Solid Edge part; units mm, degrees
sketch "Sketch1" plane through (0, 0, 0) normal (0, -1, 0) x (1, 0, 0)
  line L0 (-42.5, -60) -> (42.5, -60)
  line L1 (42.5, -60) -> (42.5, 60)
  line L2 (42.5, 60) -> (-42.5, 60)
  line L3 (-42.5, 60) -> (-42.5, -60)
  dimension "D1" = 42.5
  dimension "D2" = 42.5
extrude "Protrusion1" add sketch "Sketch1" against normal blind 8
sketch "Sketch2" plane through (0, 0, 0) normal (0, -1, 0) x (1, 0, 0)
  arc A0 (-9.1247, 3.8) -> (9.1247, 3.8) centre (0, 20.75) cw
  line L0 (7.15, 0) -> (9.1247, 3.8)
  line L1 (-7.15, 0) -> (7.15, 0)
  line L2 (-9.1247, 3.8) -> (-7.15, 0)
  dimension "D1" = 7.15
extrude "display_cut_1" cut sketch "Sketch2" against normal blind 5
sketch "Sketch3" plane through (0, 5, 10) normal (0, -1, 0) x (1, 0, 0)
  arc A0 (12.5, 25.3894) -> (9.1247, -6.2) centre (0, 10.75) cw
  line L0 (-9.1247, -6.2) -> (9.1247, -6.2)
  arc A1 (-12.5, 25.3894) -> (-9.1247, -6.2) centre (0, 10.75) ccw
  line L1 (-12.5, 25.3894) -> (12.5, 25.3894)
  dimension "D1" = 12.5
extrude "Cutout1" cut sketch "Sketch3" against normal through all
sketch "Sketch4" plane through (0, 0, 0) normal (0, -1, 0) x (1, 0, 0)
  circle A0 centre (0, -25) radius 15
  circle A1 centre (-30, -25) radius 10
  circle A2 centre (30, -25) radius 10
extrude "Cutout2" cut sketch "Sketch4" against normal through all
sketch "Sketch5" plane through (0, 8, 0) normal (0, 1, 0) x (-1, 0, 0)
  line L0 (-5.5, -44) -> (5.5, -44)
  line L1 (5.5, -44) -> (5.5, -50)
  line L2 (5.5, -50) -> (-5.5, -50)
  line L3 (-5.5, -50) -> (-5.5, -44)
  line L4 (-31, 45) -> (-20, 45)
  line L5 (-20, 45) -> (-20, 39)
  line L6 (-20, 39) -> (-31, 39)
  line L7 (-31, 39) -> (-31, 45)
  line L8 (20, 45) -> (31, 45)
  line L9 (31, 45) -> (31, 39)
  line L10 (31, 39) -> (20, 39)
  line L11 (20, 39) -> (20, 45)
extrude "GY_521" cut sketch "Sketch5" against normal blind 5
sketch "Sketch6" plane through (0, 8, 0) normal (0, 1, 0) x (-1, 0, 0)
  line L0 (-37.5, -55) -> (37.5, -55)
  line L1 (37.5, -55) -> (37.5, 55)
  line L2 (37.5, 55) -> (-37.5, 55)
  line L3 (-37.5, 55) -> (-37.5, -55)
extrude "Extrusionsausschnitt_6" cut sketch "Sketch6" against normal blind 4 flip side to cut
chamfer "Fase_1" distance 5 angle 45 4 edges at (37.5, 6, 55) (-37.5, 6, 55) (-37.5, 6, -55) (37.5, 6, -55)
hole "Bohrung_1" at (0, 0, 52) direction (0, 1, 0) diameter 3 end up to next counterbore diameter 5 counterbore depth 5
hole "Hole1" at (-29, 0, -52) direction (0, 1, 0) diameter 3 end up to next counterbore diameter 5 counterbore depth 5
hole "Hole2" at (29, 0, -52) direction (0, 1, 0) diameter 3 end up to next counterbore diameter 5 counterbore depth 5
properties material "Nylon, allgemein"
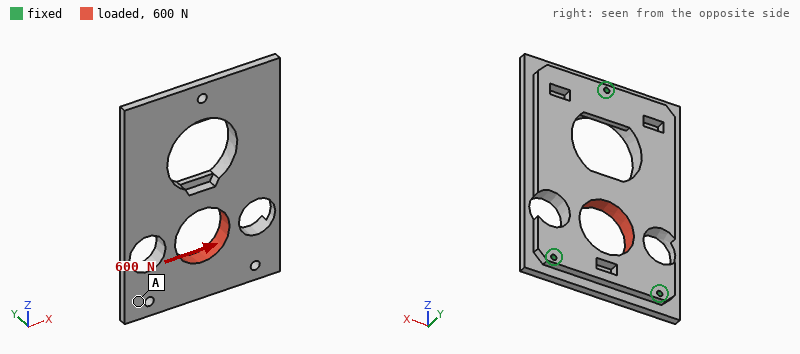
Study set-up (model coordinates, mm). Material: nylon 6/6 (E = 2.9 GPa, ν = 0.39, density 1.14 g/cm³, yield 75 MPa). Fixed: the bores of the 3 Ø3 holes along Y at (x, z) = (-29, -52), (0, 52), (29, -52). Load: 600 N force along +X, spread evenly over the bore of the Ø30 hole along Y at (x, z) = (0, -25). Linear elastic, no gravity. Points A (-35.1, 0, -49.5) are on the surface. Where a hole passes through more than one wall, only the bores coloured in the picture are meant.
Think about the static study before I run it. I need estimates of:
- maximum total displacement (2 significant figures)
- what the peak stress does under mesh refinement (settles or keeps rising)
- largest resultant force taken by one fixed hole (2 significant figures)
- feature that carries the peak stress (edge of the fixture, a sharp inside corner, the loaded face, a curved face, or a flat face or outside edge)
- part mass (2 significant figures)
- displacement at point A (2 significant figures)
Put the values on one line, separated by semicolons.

0.13 mm; keeps rising; 250 N; edge of the fixture; 60 g; 0.029 mm
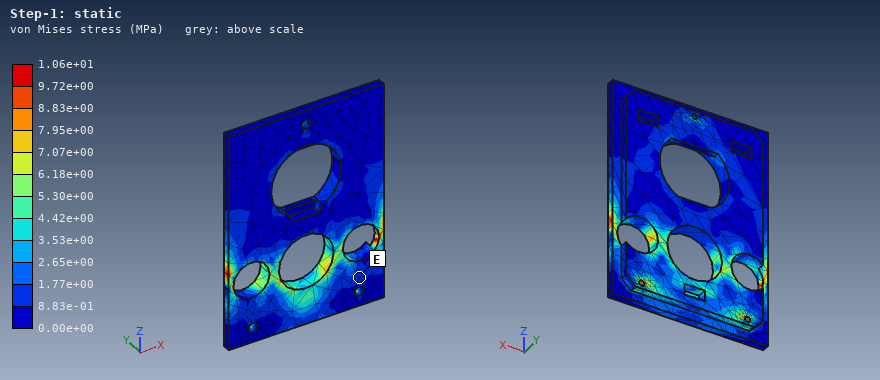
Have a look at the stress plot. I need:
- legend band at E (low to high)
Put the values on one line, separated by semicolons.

8.83e-01 to 1.77e+00 MPa
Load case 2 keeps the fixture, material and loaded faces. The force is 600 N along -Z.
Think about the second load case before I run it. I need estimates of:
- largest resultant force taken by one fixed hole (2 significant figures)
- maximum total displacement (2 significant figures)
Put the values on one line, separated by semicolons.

230 N; 0.11 mm
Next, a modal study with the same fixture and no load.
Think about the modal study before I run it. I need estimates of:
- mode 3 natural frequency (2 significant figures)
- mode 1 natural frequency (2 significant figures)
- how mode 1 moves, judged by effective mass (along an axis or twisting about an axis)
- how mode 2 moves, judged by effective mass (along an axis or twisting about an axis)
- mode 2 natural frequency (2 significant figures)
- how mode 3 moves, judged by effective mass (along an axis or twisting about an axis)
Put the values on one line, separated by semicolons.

1200 Hz; 430 Hz; twisting about Z; along Y; 570 Hz; twisting about X
